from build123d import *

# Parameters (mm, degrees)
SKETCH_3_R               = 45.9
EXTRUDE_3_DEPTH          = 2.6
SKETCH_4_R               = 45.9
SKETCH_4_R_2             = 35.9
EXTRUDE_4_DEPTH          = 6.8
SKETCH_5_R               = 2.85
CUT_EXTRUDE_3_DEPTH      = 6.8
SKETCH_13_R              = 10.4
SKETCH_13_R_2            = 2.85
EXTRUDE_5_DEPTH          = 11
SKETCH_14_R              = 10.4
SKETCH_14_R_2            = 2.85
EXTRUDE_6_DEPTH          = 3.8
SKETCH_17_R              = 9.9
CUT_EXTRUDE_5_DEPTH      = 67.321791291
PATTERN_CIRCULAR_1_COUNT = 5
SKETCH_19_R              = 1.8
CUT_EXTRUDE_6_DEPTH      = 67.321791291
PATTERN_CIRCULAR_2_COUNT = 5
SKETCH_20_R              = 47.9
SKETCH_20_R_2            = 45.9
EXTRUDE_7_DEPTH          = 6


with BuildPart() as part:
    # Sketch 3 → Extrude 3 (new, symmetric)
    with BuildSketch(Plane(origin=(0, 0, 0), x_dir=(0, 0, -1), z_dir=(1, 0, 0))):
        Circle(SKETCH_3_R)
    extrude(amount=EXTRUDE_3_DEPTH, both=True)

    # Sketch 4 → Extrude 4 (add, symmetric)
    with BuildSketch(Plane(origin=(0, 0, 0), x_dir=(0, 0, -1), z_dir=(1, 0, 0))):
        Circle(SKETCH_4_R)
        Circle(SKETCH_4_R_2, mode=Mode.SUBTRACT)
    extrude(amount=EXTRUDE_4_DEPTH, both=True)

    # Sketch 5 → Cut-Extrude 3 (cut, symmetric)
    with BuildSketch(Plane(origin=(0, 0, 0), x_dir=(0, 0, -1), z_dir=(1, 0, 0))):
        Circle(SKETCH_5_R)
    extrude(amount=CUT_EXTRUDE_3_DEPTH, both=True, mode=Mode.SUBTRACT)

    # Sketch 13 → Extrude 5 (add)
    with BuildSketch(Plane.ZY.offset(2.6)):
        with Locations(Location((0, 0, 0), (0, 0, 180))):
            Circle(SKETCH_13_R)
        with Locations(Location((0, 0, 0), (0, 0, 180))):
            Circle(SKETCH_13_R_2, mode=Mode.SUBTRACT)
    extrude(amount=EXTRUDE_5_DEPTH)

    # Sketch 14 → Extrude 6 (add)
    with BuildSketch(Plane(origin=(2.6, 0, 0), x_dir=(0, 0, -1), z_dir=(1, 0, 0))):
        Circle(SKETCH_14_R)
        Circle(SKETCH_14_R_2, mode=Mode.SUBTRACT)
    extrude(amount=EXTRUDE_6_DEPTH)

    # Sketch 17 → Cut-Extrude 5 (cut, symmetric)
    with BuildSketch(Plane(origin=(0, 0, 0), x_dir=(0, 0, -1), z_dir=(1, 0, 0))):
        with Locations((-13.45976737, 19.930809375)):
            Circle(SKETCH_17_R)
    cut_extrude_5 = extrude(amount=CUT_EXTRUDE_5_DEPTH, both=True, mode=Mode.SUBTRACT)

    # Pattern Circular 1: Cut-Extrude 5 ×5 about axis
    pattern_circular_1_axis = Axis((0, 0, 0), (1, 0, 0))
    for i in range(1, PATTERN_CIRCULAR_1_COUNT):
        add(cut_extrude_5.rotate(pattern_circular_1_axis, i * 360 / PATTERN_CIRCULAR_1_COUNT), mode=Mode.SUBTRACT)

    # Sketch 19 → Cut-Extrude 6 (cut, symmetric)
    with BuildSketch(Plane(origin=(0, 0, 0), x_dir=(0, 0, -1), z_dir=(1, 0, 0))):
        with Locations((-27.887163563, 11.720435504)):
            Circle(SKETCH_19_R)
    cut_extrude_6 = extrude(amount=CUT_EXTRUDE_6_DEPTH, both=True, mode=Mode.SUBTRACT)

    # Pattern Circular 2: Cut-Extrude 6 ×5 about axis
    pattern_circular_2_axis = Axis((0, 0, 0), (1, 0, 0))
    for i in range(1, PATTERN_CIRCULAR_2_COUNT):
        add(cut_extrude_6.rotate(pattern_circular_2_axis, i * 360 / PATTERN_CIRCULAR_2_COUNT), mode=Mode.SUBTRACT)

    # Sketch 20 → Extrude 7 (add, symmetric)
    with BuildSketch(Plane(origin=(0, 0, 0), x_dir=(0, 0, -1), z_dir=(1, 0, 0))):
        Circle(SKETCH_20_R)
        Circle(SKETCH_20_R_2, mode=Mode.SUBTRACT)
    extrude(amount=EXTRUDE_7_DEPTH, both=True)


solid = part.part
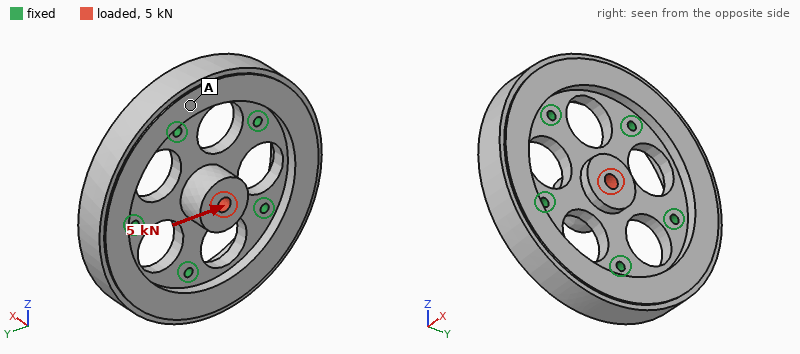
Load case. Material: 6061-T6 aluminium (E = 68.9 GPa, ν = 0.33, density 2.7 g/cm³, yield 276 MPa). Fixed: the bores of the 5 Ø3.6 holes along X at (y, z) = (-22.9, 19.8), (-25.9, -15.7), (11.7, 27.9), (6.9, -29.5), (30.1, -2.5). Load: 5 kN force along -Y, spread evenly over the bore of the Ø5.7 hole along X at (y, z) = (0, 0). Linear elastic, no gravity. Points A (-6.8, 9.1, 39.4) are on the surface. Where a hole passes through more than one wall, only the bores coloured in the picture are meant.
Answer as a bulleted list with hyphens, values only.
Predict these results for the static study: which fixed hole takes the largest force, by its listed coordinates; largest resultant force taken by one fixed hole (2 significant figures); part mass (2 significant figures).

- (30.1, -2.5)
- 1.6 kN
- 160 g
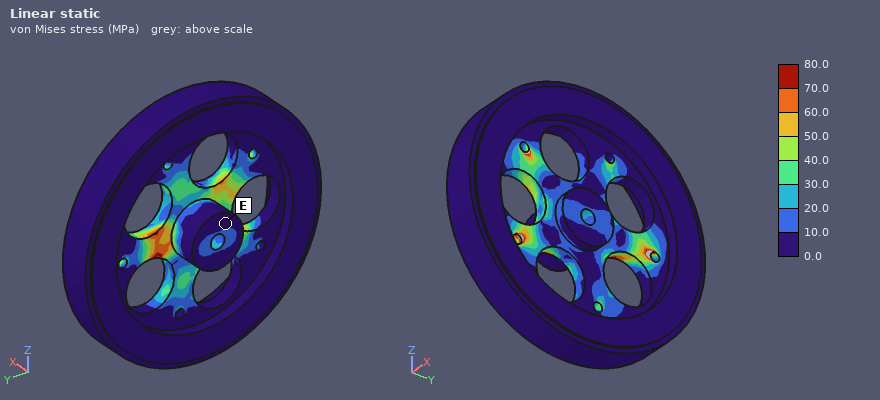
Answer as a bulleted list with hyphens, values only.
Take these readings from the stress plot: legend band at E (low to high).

- 0.0 to 10.0 MPa
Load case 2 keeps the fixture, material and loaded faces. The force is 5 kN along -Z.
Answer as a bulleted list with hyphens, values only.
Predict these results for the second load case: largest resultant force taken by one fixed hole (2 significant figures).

- 1.6 kN
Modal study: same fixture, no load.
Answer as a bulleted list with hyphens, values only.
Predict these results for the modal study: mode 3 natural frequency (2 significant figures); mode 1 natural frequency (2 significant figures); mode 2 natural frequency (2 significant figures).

- 7200 Hz
- 7000 Hz
- 7000 Hz
